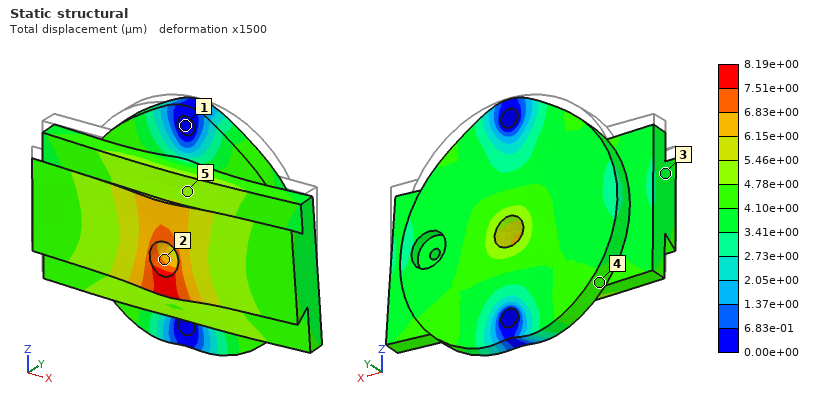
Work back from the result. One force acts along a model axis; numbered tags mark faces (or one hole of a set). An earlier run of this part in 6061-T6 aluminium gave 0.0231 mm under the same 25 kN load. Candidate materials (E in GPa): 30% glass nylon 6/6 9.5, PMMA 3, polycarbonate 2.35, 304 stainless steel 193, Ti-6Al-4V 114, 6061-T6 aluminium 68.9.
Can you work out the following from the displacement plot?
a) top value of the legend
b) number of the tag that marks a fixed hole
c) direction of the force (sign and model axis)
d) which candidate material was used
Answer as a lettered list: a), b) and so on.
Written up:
a) 8.19e+00 µm
b) 1
c) -Z
d) 304 stainless steel
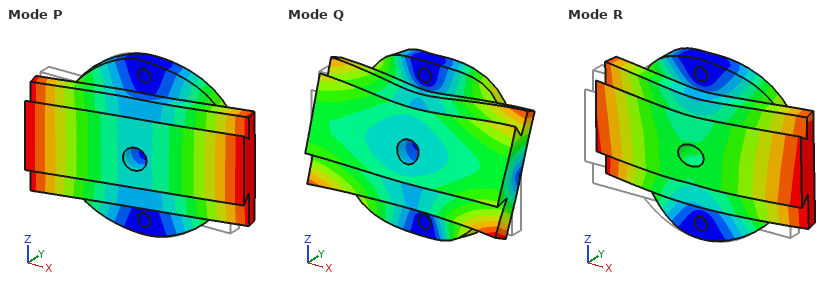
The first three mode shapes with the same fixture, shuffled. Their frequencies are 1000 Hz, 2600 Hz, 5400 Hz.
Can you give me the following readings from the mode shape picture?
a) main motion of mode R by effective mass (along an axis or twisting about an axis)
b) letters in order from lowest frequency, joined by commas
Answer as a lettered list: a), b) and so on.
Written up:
a) along Y
b) P, R, Q
